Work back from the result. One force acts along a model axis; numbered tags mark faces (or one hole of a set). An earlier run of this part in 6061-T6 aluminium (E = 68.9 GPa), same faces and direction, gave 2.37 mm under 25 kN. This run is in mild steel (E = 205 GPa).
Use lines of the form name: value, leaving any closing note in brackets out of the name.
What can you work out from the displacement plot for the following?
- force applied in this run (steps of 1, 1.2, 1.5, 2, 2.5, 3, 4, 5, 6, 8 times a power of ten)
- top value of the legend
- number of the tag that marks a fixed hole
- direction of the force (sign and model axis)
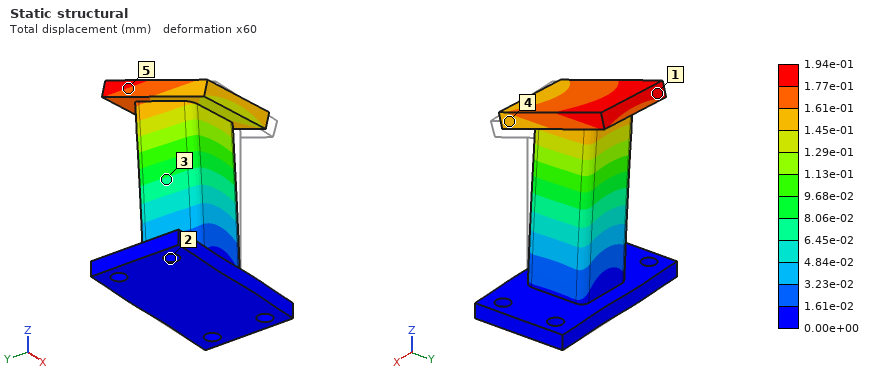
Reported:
force applied in this run: 6 kN
top value of the legend: 1.94e-01 mm
number of the tag that marks a fixed hole: 2
direction of the force: -X
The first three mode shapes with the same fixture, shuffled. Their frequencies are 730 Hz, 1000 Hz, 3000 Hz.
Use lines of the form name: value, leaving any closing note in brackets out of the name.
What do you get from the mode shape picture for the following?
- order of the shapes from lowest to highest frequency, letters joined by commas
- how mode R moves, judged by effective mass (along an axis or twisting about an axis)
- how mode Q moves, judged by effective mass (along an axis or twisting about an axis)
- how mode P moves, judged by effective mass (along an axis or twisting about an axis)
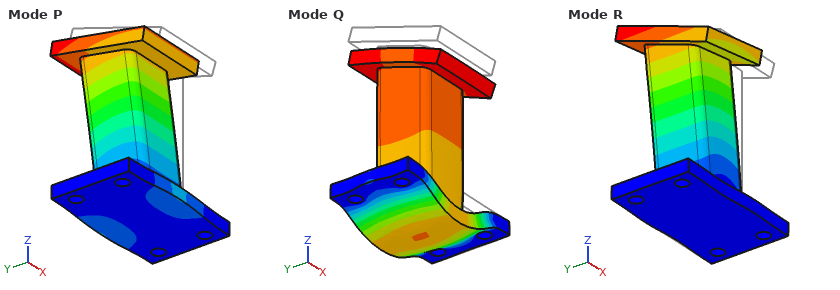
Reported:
order of the shapes from lowest to highest frequency, letters joined by commas: P, R, Q
how mode R moves, judged by effective mass: along X
how mode Q moves, judged by effective mass: along Z
how mode P moves, judged by effective mass: along Y
